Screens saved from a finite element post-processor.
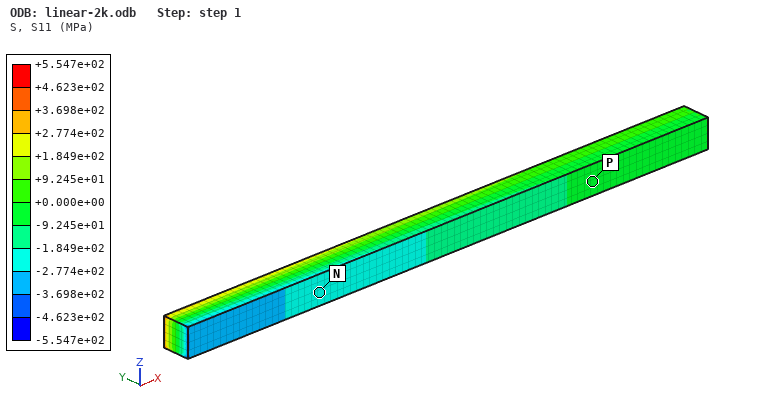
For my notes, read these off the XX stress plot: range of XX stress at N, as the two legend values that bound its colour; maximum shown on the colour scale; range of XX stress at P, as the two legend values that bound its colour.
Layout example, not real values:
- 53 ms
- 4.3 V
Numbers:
- -2.774e+02 to -1.849e+02 MPa
- +5.547e+02 MPa
- -9.245e+01 to +0.000e+00 MPa
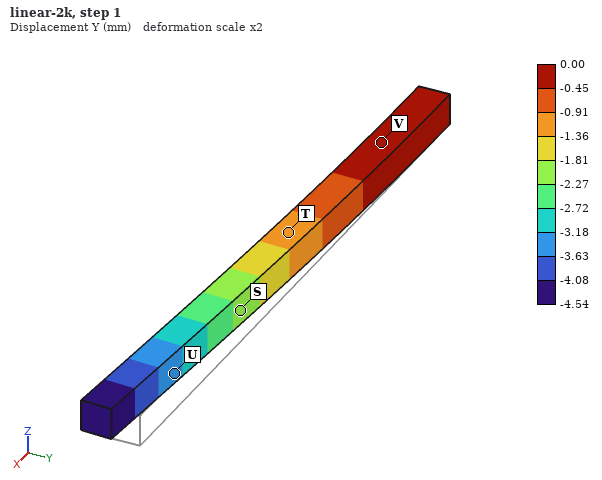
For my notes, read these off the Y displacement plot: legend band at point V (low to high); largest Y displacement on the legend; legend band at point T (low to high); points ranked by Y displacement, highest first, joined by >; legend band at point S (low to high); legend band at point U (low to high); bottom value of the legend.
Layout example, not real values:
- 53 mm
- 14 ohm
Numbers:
- -0.45 to 0.00 mm
- 0.00 mm
- -1.36 to -0.91 mm
- V > T > S > U
- -2.27 to -1.81 mm
- -3.63 to -3.18 mm
- -4.54 mm
